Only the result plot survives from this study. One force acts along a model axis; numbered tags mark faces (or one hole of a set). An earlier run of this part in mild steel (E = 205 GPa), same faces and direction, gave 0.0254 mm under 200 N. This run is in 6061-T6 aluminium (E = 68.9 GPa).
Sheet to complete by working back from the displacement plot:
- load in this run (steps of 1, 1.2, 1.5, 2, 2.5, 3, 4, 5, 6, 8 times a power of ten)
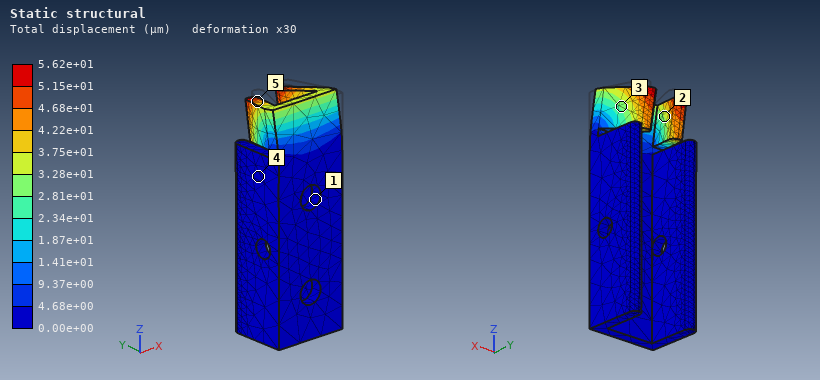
150 N
